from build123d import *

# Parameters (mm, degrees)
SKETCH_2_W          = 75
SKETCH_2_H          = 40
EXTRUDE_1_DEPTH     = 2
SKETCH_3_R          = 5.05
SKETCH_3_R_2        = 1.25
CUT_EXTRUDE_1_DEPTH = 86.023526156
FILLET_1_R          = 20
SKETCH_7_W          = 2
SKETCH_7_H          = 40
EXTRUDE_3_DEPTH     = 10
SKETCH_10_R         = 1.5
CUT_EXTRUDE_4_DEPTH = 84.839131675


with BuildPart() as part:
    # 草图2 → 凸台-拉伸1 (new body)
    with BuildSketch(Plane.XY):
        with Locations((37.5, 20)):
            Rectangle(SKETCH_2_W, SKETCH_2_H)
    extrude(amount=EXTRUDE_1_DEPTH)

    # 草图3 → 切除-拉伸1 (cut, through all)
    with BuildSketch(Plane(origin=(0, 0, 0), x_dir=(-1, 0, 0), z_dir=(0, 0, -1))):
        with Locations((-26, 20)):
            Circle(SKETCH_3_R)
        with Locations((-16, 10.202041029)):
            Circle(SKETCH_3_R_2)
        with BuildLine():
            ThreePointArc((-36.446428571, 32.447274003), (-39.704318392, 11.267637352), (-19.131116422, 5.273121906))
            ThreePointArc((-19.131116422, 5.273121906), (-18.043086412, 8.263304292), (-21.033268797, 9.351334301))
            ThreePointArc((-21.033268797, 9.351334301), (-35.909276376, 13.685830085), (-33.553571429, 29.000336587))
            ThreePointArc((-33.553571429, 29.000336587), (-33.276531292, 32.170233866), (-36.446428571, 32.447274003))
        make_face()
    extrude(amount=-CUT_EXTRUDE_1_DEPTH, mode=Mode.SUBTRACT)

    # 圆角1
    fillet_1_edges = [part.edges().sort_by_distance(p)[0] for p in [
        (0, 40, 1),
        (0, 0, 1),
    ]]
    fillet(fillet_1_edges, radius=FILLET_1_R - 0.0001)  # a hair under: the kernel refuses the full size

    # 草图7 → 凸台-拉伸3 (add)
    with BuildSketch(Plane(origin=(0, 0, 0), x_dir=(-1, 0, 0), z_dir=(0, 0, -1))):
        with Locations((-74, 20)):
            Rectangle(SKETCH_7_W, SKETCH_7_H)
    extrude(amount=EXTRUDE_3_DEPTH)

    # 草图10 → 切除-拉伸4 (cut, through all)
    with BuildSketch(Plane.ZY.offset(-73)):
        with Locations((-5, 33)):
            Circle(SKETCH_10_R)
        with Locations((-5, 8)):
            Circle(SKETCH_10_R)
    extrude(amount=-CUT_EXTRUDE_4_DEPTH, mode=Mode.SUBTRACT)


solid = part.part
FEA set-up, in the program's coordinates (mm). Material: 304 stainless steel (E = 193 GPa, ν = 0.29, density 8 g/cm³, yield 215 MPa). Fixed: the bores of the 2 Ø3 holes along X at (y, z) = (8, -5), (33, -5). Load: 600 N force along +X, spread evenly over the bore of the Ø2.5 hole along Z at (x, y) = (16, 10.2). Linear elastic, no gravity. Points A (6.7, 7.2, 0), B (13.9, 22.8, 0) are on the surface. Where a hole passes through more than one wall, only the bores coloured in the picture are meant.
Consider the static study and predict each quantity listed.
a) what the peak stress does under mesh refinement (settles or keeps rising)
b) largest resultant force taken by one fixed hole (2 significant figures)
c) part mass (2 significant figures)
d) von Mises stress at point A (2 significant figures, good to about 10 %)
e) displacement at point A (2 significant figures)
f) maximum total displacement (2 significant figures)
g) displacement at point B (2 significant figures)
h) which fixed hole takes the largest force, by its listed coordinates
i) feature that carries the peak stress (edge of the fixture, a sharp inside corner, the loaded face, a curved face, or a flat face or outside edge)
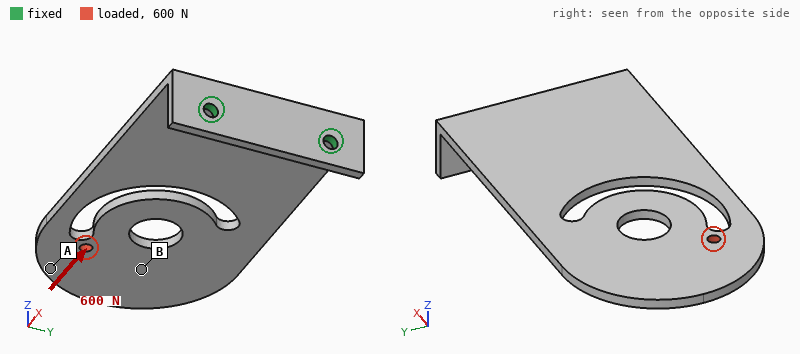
keeps rising
530 N
47 g
30 MPa
0.18 mm
0.19 mm
0.14 mm
(8, -5)
edge of the fixture
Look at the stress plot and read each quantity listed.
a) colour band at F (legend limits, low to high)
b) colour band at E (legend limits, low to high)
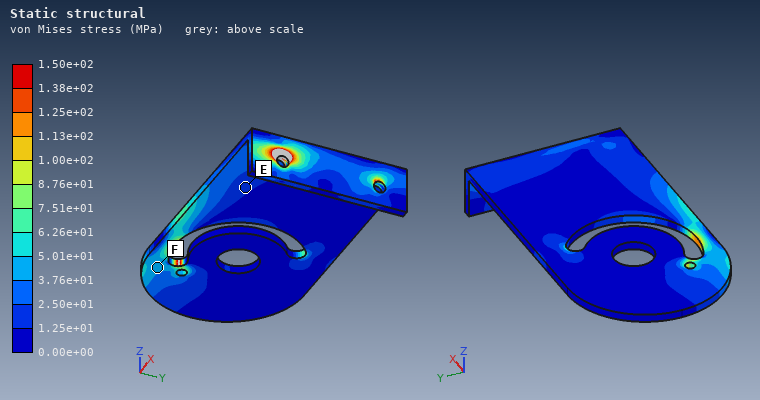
3.76e+01 to 5.01e+01 MPa
1.25e+01 to 2.50e+01 MPa
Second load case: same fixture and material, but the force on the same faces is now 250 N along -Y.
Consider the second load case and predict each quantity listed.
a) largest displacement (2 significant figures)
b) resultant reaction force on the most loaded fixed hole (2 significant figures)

0.11 mm
560 N
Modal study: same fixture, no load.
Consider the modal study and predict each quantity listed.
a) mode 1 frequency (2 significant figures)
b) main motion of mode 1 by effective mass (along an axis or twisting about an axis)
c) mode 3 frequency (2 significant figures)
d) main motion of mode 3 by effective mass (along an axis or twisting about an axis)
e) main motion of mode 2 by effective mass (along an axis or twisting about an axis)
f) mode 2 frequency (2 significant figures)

280 Hz
along Z
1400 Hz
along Z
twisting about X
1100 Hz
